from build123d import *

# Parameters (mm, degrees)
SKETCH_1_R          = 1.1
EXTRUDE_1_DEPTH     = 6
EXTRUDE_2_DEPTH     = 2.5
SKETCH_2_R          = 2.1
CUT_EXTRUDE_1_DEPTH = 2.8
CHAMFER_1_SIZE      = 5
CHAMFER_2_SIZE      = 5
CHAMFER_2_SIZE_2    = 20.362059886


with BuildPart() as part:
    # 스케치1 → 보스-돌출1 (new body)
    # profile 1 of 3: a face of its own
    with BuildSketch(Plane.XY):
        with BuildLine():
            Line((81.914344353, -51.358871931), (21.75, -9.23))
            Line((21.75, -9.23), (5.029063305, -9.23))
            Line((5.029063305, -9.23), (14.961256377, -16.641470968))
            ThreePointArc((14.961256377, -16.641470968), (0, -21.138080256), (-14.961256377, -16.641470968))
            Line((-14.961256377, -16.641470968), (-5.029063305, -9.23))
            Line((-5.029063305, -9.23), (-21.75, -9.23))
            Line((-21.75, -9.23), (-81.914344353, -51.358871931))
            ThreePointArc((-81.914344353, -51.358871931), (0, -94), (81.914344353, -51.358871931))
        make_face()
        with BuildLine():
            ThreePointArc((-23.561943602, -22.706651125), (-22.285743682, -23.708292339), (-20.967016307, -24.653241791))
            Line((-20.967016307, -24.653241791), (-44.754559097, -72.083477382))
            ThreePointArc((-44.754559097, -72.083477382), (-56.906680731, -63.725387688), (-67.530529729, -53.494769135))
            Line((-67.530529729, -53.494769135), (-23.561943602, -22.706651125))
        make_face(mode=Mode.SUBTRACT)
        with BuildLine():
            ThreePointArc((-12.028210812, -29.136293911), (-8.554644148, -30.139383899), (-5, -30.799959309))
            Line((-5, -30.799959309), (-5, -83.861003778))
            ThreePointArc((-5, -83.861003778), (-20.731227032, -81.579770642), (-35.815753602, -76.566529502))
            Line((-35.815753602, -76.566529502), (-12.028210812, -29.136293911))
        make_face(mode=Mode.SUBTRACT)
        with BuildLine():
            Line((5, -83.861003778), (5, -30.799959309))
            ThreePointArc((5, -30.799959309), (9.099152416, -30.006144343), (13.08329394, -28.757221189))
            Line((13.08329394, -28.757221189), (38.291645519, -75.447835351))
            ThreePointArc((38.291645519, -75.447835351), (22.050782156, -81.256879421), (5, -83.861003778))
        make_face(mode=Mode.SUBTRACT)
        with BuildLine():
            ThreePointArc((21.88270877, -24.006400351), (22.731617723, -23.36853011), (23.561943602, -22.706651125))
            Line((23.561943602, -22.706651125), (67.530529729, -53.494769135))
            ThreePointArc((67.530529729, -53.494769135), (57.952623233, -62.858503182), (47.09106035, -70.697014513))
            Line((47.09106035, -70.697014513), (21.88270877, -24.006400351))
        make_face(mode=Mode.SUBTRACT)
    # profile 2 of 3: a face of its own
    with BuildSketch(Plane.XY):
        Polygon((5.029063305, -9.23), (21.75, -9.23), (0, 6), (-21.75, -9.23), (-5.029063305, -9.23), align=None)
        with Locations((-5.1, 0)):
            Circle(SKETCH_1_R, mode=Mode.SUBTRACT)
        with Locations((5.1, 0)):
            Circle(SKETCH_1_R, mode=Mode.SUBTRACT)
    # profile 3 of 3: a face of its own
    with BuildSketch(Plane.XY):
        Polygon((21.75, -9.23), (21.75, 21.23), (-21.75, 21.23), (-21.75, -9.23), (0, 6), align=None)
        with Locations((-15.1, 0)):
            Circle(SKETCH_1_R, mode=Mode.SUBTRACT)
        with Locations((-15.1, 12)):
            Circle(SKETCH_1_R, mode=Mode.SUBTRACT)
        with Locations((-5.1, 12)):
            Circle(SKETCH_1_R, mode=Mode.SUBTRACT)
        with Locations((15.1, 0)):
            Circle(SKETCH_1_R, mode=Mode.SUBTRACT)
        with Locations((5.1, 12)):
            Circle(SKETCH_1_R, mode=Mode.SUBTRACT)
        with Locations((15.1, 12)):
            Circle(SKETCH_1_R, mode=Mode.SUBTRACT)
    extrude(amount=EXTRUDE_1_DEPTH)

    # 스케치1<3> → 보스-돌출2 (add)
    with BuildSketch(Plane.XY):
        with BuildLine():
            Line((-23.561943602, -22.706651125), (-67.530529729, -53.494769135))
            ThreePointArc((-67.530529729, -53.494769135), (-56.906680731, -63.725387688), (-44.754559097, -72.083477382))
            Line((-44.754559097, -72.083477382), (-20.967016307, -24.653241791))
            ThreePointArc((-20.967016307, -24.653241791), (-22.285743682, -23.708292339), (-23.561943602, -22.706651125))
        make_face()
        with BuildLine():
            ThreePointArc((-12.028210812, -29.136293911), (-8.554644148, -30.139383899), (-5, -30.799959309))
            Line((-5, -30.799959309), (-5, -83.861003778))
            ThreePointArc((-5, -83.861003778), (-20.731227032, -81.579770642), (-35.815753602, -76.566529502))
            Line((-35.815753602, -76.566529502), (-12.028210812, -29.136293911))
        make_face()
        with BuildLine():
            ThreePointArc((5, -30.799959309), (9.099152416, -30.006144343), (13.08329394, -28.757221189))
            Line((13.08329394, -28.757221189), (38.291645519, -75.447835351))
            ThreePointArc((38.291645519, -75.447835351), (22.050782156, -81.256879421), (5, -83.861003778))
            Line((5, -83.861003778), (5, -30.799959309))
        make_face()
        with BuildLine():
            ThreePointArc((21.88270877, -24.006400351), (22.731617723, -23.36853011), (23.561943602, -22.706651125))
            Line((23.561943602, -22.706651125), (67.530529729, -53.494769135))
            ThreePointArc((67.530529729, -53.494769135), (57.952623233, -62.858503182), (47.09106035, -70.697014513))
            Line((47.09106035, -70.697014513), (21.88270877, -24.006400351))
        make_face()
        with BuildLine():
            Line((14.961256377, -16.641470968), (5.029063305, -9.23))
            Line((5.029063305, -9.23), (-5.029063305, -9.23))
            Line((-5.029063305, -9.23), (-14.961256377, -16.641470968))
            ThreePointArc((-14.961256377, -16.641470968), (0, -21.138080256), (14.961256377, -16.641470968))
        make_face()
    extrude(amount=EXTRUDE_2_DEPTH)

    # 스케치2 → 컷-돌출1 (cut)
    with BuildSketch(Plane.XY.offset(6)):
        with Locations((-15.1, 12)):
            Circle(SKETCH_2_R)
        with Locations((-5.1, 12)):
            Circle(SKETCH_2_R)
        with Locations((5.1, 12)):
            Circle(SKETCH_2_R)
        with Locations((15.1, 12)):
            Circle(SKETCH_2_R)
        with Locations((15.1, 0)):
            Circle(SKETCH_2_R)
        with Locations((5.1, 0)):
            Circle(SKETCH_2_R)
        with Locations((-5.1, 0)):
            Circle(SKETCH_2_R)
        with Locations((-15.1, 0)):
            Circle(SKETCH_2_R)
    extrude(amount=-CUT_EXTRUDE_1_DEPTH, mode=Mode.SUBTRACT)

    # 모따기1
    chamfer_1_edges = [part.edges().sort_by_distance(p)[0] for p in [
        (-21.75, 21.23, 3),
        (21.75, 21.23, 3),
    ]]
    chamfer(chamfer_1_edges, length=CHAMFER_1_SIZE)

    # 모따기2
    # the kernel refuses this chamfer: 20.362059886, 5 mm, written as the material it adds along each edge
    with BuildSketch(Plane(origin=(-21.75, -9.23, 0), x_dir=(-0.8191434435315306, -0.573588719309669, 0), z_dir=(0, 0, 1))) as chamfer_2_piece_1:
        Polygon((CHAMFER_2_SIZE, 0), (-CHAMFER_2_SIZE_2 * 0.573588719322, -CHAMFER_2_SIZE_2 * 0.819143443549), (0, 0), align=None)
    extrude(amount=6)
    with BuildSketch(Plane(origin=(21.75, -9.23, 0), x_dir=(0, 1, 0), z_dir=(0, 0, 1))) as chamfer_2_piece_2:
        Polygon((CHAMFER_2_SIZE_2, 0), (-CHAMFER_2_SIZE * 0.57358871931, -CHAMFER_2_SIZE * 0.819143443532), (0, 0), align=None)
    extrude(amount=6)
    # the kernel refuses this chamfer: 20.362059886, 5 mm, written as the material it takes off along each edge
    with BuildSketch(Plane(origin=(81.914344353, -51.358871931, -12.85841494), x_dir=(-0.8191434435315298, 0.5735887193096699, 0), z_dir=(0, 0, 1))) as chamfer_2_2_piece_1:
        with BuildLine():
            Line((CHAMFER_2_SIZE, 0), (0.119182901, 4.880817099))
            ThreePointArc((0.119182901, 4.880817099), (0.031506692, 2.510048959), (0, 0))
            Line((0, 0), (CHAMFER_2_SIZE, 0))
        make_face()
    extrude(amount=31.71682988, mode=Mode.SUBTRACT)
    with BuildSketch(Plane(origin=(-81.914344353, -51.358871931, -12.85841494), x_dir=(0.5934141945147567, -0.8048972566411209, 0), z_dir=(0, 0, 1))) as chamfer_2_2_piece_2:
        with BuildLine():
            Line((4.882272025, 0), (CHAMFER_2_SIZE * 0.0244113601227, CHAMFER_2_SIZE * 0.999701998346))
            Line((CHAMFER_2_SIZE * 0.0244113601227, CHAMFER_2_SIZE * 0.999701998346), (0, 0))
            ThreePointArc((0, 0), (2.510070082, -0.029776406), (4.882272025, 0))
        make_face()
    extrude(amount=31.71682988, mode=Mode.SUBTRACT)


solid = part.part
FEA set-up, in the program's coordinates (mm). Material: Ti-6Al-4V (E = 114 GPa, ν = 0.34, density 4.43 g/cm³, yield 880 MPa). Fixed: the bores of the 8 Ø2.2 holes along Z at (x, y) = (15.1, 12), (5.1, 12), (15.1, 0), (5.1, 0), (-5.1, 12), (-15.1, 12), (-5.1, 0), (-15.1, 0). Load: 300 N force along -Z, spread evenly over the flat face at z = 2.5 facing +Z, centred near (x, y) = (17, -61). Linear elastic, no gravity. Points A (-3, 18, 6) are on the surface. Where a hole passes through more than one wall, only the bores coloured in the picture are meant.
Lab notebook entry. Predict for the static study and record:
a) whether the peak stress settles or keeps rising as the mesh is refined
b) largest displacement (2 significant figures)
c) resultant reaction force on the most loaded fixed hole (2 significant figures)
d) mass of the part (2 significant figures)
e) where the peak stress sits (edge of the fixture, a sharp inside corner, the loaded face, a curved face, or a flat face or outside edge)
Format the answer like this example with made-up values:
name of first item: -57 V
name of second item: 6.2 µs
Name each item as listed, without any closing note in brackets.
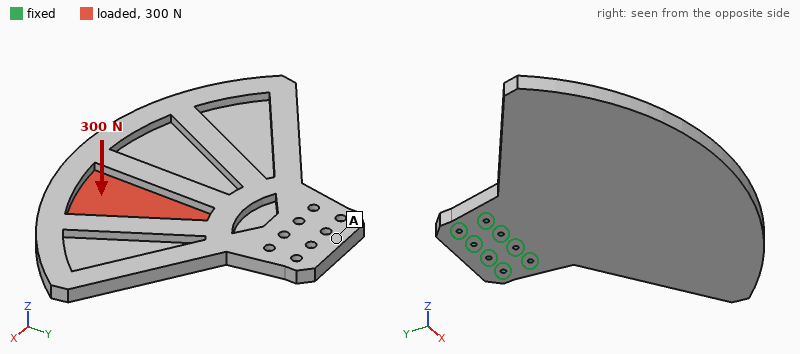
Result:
whether the peak stress settles or keeps rising as the mesh is refined: keeps rising
largest displacement: 0.56 mm
resultant reaction force on the most loaded fixed hole: 630 N
mass of the part: 220 g
where the peak stress sits: edge of the fixture
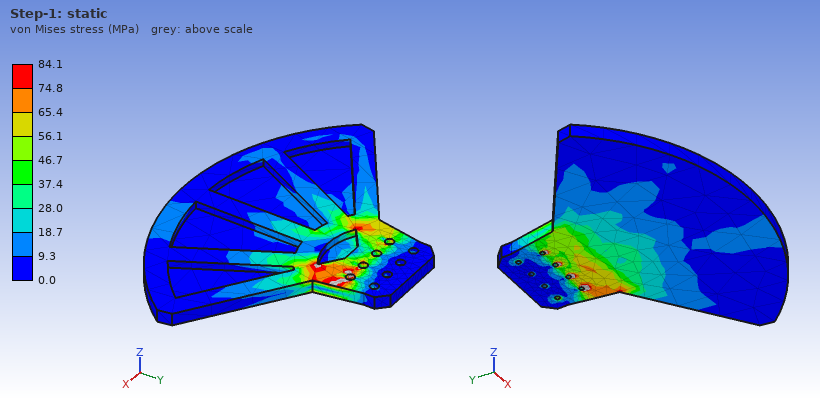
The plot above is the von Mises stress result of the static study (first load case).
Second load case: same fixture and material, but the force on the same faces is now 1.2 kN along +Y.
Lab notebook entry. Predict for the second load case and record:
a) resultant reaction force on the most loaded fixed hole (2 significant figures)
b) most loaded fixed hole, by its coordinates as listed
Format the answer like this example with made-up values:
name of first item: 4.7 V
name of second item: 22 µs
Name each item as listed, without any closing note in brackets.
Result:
resultant reaction force on the most loaded fixed hole: 660 N
most loaded fixed hole, by its coordinates as listed: (15.1, 0)
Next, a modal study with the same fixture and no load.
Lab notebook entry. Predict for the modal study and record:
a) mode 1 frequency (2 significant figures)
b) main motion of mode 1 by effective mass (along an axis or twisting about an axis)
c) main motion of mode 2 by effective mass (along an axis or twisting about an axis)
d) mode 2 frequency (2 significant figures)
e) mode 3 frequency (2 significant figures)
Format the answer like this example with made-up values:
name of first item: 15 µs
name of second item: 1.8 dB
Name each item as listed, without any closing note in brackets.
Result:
mode 1 frequency: 390 Hz
main motion of mode 1 by effective mass: along Z
main motion of mode 2 by effective mass: twisting about Y
mode 2 frequency: 580 Hz
mode 3 frequency: 1300 Hz
